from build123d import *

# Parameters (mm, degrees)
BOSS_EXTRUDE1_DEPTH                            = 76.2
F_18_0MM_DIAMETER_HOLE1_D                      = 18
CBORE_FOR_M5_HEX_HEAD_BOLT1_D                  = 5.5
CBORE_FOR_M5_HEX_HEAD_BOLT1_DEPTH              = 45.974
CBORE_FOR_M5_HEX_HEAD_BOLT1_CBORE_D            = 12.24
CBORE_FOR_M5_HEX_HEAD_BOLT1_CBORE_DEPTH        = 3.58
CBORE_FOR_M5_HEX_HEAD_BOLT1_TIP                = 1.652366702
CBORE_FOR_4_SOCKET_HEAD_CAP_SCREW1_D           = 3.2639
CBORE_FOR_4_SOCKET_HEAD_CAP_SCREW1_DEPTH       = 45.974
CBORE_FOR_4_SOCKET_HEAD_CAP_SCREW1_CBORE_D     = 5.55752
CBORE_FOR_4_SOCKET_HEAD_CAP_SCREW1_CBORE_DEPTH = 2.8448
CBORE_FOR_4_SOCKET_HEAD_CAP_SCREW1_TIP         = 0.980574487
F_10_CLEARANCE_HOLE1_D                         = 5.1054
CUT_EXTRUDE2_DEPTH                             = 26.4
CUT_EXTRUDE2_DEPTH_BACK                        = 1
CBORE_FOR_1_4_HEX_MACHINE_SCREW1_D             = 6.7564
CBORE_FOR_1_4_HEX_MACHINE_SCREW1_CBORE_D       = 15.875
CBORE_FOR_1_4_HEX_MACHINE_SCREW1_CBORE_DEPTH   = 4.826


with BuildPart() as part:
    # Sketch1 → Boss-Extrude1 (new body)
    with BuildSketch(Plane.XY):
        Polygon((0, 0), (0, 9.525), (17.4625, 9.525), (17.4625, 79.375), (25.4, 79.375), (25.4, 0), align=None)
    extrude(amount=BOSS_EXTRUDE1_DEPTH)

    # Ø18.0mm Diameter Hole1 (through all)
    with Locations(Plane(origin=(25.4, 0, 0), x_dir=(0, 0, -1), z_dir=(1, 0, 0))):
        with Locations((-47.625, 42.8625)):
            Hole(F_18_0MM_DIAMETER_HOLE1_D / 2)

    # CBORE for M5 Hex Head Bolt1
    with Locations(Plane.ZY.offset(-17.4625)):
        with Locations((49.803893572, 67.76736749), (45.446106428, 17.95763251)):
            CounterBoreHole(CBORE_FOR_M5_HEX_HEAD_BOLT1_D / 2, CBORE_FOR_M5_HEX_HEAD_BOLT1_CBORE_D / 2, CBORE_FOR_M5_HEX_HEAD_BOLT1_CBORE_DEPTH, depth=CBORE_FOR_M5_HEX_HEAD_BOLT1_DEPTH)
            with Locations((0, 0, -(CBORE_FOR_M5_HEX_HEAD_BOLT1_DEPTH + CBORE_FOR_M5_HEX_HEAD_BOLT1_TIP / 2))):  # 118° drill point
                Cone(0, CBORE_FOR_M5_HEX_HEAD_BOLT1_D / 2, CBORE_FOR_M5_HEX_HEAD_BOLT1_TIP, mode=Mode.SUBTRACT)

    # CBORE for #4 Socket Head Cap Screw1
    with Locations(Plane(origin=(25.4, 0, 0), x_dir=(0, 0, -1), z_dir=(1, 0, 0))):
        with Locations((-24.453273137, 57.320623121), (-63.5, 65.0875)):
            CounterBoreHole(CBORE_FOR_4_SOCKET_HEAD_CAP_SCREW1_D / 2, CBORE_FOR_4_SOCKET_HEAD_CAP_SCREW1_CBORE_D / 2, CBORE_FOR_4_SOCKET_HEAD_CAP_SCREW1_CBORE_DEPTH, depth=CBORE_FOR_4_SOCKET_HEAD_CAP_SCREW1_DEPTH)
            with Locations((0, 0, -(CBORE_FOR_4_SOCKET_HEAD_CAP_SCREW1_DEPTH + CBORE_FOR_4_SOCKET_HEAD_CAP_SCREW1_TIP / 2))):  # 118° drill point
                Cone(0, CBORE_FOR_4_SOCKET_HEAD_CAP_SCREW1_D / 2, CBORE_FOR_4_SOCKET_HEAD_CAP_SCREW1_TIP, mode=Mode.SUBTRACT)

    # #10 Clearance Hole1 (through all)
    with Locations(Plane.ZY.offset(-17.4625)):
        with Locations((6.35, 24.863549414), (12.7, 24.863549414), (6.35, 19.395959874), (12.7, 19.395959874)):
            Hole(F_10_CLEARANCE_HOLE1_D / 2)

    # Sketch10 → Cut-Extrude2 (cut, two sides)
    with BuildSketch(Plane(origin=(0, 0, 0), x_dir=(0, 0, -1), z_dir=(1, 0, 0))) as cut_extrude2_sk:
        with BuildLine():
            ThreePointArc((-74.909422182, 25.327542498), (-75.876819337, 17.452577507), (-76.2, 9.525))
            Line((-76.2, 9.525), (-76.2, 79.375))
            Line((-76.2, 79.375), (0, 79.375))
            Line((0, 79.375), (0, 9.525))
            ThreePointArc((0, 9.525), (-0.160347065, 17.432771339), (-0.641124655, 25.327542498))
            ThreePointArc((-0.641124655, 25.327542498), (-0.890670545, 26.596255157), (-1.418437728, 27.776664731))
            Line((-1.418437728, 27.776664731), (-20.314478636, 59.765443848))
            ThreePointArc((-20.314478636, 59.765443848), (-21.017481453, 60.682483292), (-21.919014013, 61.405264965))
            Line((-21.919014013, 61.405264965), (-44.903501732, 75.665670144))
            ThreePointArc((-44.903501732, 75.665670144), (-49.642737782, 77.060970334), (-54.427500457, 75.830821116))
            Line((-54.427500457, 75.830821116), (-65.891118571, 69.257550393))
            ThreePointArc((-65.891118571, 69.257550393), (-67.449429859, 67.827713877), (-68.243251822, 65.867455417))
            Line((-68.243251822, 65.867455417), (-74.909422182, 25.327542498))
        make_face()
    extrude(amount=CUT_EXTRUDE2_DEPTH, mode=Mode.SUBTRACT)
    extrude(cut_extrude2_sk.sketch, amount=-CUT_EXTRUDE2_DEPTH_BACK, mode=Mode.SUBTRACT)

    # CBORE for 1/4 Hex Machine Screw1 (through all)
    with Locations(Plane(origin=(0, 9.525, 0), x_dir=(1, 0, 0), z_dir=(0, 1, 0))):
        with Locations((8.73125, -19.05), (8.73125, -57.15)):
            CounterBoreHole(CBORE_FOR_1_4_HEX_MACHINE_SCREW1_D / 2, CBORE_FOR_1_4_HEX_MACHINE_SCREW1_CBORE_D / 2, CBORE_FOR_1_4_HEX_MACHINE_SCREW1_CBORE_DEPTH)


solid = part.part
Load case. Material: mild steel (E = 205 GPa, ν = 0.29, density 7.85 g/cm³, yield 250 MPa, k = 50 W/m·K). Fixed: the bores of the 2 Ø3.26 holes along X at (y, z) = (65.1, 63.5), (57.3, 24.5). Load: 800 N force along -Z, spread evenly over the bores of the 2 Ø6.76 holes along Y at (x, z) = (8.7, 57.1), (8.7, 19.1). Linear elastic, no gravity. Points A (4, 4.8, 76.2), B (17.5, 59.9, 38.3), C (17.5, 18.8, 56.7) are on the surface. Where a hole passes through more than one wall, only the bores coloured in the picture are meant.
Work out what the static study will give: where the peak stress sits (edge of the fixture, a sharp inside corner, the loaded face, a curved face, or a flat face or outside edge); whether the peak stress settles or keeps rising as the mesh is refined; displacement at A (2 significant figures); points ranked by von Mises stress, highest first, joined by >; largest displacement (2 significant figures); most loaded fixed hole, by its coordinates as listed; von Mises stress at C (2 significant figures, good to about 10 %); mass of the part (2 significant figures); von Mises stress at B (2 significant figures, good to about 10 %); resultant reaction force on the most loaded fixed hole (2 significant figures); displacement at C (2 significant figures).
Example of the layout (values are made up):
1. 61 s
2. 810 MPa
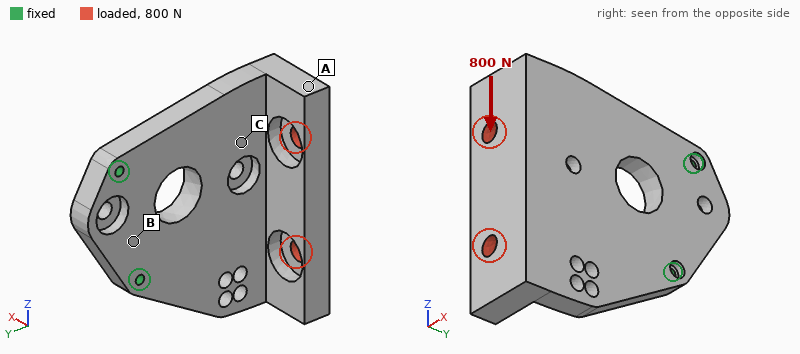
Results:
1. edge of the fixture
2. keeps rising
3. 34 µm
4. C > B > A
5. 37 µm
6. (57.3, 24.5)
7. 18 MPa
8. 340 g
9. 11 MPa
10. 1.3 kN
11. 15 µm
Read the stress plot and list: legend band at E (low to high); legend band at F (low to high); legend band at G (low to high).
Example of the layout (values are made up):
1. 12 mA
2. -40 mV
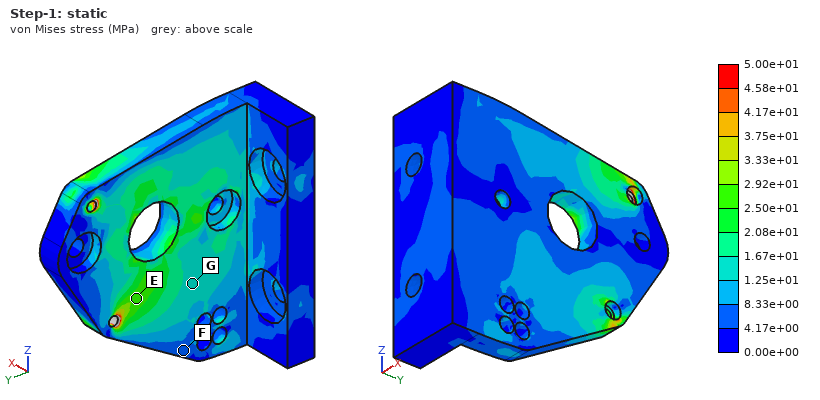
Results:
1. 2.50e+01 to 2.92e+01 MPa
2. 4.17e+00 to 8.33e+00 MPa
3. 1.25e+01 to 1.67e+01 MPa
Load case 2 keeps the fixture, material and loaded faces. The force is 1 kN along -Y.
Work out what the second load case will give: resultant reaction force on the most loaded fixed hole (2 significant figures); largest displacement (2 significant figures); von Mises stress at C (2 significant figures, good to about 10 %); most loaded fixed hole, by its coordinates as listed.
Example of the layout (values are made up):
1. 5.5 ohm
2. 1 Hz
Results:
1. 650 N
2. 91 µm
3. 21 MPa
4. (57.3, 24.5)
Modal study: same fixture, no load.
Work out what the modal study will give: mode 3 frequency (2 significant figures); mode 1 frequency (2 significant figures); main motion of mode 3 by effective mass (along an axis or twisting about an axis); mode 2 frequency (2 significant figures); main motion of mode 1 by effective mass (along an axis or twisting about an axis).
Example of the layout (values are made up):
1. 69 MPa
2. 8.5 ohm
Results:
1. 4000 Hz
2. 750 Hz
3. along Z
4. 1900 Hz
5. along X
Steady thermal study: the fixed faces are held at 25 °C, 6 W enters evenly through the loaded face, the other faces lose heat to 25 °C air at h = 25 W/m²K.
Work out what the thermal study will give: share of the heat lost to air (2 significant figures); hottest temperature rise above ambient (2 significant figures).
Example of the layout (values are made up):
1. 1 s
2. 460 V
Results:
1. 48 %
2. 15 K
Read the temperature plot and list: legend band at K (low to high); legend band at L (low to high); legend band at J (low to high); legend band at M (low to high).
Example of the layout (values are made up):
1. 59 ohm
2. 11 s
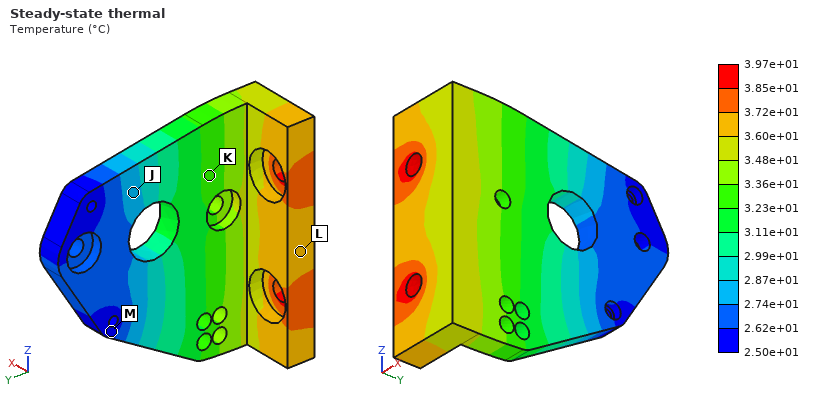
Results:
1. 3.23e+01 to 3.36e+01 °C
2. 3.60e+01 to 3.72e+01 °C
3. 2.74e+01 to 2.87e+01 °C
4. 2.50e+01 to 2.62e+01 °C
